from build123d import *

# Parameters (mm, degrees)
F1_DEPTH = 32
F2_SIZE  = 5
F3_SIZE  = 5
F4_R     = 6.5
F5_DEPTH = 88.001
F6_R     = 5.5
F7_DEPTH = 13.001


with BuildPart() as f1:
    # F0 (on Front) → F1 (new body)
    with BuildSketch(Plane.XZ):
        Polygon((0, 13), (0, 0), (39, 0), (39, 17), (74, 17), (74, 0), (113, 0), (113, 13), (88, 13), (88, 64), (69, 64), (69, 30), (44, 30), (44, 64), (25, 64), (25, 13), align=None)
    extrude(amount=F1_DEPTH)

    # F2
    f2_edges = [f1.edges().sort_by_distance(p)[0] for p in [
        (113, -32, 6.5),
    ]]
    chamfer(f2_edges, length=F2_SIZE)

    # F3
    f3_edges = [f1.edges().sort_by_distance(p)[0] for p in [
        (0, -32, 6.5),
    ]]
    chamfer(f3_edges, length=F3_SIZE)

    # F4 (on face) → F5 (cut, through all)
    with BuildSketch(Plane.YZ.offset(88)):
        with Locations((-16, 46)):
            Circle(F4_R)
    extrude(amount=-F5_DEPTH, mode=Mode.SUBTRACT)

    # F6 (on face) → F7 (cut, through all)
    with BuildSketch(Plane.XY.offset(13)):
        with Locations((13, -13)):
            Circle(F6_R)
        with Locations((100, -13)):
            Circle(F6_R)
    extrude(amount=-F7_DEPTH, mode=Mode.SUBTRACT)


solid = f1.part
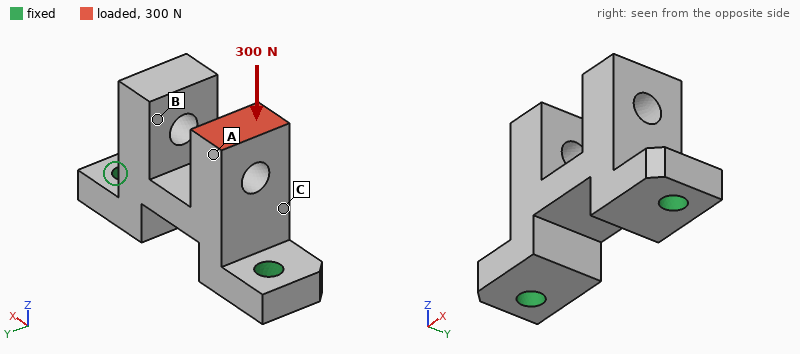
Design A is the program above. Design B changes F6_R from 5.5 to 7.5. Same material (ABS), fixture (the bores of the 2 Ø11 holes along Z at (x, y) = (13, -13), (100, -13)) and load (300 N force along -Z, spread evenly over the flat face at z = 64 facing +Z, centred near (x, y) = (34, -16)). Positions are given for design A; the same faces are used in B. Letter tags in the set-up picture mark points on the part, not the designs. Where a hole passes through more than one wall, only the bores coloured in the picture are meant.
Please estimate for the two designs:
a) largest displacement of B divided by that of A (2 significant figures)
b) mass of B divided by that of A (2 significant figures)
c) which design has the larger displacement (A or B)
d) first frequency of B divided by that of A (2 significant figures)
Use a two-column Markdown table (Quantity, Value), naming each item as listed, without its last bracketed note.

| Quantity | Value |
|---|---|
| largest displacement of B divided by that of A | 0.82 |
| mass of B divided by that of A | 0.98 |
| which design has the larger displacement | A |
| first frequency of B divided by that of A | 1.1 |
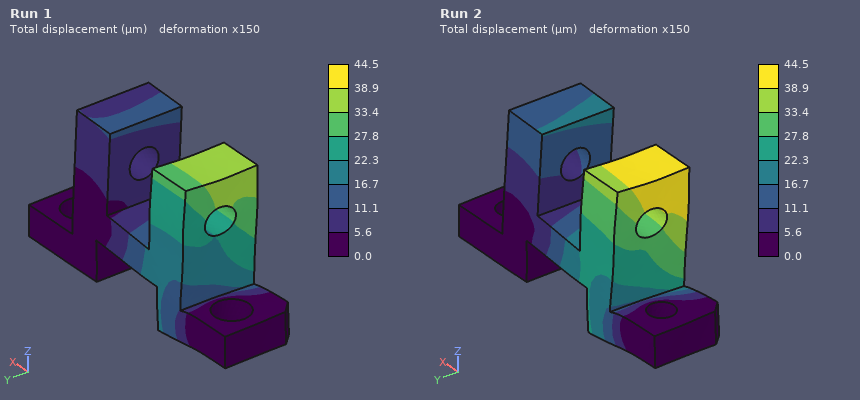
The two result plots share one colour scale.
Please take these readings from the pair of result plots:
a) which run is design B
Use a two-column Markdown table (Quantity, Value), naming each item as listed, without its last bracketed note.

| Quantity | Value |
|---|---|
| which run is design B | Run 1 |
